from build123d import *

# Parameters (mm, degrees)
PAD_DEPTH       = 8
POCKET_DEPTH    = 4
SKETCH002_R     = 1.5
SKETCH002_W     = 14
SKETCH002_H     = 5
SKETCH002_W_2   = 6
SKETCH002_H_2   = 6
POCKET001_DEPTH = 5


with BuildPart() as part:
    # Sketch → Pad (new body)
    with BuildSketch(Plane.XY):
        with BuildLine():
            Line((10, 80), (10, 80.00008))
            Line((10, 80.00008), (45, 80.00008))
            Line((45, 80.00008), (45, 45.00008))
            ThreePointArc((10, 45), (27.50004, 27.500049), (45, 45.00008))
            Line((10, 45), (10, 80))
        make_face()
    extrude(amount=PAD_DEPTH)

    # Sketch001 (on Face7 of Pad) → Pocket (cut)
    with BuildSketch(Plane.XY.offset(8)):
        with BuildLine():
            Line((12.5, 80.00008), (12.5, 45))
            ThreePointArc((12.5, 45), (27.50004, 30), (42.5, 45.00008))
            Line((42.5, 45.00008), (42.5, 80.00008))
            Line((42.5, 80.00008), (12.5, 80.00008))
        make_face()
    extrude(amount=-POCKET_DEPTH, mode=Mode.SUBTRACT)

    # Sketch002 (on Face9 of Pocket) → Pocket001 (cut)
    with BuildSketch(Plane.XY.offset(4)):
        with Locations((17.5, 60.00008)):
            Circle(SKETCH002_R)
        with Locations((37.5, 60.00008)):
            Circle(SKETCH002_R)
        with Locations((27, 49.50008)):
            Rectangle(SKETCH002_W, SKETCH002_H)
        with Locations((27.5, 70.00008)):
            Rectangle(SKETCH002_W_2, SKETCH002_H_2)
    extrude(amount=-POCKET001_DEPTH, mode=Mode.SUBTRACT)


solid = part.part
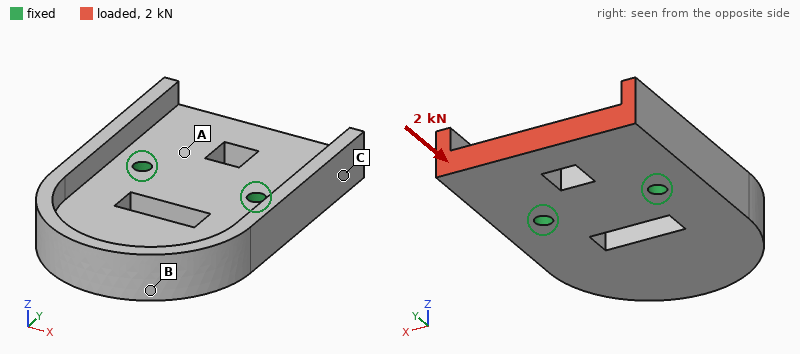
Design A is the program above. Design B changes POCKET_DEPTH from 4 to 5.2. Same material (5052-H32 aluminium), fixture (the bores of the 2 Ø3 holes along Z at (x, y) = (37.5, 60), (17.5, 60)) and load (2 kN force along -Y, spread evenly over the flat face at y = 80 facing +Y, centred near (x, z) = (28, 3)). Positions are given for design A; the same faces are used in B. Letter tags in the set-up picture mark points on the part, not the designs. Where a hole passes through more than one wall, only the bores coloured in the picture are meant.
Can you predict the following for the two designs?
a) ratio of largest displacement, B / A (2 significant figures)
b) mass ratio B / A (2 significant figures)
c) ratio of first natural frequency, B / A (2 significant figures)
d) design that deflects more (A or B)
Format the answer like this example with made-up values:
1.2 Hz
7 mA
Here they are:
3.6
0.80
0.78
B
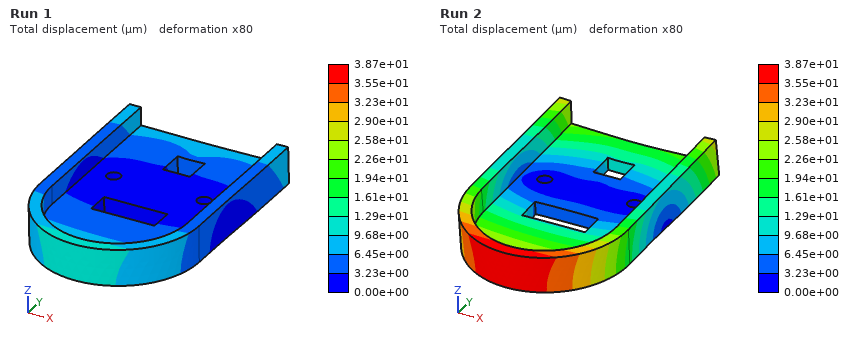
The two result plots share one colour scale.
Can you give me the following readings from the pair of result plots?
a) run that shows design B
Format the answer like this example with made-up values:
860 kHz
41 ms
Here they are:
Run 2
